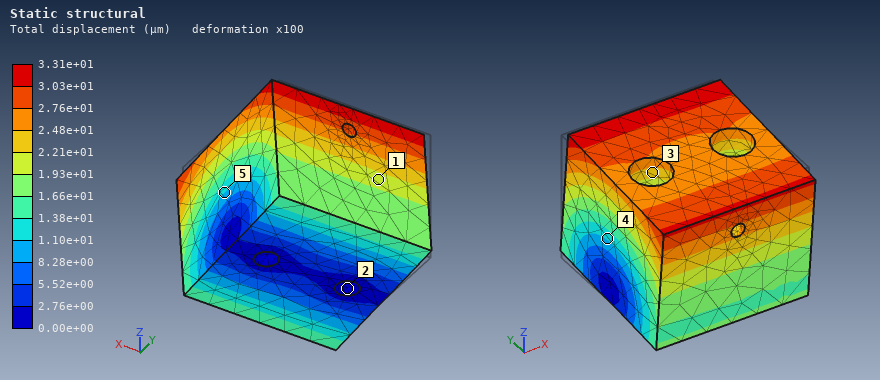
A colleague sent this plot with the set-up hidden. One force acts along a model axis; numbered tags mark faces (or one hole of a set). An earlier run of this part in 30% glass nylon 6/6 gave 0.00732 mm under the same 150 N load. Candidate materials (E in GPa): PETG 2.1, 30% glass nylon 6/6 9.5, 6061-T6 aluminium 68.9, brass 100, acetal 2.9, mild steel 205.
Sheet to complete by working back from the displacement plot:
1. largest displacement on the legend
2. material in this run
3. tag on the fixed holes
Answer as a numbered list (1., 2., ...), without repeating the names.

1. 3.31e+01 µm
2. PETG
3. 2
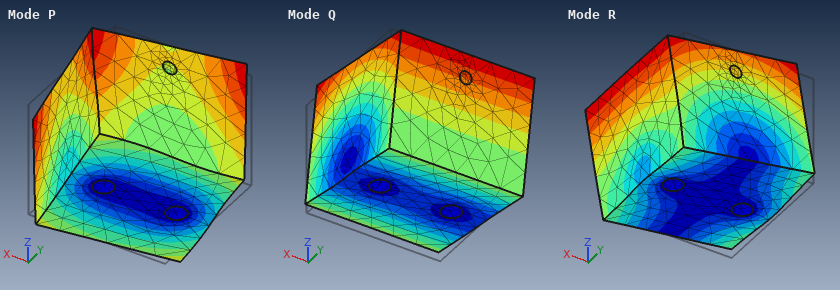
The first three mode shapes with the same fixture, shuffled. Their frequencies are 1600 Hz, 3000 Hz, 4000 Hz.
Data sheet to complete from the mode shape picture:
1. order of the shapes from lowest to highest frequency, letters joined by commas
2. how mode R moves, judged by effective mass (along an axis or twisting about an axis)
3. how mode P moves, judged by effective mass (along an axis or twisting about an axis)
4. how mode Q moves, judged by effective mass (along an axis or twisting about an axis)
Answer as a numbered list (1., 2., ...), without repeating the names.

1. Q, R, P
2. along X
3. twisting about Z
4. along Y
